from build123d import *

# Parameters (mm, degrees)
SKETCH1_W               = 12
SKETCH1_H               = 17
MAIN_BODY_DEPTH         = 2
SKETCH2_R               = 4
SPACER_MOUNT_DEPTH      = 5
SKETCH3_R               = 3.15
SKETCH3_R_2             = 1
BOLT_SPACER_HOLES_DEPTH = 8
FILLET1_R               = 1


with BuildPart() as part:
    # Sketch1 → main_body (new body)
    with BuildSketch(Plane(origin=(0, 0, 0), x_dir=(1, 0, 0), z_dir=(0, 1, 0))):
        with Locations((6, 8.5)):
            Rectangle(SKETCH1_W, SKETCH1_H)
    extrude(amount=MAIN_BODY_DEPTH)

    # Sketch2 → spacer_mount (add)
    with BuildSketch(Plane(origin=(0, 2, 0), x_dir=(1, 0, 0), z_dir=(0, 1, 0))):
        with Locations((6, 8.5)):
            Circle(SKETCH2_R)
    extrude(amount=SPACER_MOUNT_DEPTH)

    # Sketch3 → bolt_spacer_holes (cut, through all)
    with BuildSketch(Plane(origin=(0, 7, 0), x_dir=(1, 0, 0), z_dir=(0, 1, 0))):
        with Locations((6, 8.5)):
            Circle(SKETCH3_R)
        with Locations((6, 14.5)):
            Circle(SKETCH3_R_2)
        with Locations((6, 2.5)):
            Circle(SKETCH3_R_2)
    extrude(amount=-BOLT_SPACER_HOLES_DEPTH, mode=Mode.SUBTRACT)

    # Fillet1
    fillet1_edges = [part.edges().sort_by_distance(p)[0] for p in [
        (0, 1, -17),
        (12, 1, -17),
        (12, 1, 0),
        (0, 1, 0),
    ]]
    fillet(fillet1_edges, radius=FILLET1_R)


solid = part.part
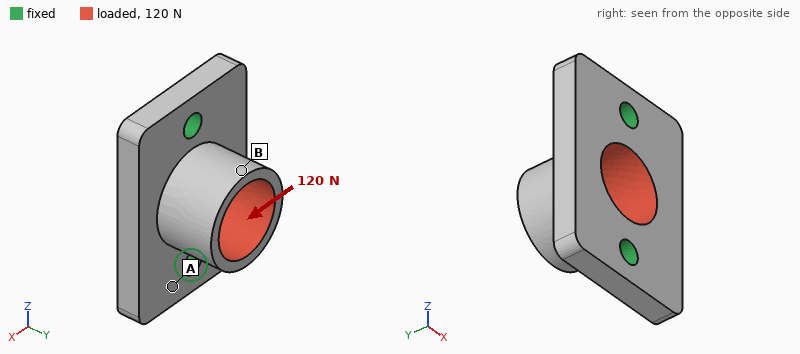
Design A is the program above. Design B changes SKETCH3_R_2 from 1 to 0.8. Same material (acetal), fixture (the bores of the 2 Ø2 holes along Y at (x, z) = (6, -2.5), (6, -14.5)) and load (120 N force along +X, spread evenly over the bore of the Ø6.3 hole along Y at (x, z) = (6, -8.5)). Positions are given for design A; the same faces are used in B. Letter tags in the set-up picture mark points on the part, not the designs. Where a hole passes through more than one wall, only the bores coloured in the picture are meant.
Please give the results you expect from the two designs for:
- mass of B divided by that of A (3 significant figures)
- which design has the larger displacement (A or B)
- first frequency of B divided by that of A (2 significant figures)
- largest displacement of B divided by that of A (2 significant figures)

1.01
B
0.91
1.1
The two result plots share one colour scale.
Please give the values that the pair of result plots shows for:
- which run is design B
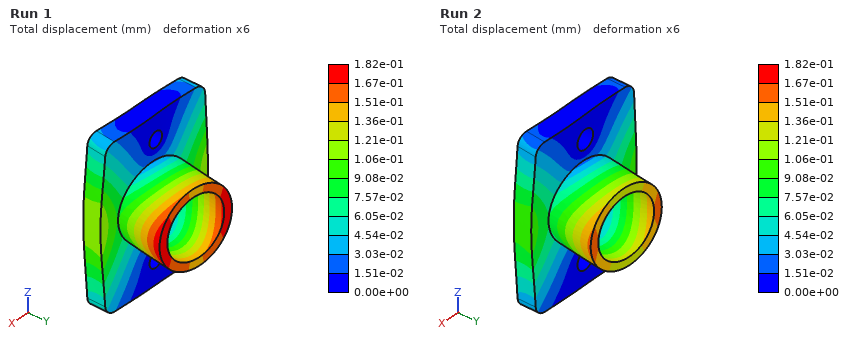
Run 1
